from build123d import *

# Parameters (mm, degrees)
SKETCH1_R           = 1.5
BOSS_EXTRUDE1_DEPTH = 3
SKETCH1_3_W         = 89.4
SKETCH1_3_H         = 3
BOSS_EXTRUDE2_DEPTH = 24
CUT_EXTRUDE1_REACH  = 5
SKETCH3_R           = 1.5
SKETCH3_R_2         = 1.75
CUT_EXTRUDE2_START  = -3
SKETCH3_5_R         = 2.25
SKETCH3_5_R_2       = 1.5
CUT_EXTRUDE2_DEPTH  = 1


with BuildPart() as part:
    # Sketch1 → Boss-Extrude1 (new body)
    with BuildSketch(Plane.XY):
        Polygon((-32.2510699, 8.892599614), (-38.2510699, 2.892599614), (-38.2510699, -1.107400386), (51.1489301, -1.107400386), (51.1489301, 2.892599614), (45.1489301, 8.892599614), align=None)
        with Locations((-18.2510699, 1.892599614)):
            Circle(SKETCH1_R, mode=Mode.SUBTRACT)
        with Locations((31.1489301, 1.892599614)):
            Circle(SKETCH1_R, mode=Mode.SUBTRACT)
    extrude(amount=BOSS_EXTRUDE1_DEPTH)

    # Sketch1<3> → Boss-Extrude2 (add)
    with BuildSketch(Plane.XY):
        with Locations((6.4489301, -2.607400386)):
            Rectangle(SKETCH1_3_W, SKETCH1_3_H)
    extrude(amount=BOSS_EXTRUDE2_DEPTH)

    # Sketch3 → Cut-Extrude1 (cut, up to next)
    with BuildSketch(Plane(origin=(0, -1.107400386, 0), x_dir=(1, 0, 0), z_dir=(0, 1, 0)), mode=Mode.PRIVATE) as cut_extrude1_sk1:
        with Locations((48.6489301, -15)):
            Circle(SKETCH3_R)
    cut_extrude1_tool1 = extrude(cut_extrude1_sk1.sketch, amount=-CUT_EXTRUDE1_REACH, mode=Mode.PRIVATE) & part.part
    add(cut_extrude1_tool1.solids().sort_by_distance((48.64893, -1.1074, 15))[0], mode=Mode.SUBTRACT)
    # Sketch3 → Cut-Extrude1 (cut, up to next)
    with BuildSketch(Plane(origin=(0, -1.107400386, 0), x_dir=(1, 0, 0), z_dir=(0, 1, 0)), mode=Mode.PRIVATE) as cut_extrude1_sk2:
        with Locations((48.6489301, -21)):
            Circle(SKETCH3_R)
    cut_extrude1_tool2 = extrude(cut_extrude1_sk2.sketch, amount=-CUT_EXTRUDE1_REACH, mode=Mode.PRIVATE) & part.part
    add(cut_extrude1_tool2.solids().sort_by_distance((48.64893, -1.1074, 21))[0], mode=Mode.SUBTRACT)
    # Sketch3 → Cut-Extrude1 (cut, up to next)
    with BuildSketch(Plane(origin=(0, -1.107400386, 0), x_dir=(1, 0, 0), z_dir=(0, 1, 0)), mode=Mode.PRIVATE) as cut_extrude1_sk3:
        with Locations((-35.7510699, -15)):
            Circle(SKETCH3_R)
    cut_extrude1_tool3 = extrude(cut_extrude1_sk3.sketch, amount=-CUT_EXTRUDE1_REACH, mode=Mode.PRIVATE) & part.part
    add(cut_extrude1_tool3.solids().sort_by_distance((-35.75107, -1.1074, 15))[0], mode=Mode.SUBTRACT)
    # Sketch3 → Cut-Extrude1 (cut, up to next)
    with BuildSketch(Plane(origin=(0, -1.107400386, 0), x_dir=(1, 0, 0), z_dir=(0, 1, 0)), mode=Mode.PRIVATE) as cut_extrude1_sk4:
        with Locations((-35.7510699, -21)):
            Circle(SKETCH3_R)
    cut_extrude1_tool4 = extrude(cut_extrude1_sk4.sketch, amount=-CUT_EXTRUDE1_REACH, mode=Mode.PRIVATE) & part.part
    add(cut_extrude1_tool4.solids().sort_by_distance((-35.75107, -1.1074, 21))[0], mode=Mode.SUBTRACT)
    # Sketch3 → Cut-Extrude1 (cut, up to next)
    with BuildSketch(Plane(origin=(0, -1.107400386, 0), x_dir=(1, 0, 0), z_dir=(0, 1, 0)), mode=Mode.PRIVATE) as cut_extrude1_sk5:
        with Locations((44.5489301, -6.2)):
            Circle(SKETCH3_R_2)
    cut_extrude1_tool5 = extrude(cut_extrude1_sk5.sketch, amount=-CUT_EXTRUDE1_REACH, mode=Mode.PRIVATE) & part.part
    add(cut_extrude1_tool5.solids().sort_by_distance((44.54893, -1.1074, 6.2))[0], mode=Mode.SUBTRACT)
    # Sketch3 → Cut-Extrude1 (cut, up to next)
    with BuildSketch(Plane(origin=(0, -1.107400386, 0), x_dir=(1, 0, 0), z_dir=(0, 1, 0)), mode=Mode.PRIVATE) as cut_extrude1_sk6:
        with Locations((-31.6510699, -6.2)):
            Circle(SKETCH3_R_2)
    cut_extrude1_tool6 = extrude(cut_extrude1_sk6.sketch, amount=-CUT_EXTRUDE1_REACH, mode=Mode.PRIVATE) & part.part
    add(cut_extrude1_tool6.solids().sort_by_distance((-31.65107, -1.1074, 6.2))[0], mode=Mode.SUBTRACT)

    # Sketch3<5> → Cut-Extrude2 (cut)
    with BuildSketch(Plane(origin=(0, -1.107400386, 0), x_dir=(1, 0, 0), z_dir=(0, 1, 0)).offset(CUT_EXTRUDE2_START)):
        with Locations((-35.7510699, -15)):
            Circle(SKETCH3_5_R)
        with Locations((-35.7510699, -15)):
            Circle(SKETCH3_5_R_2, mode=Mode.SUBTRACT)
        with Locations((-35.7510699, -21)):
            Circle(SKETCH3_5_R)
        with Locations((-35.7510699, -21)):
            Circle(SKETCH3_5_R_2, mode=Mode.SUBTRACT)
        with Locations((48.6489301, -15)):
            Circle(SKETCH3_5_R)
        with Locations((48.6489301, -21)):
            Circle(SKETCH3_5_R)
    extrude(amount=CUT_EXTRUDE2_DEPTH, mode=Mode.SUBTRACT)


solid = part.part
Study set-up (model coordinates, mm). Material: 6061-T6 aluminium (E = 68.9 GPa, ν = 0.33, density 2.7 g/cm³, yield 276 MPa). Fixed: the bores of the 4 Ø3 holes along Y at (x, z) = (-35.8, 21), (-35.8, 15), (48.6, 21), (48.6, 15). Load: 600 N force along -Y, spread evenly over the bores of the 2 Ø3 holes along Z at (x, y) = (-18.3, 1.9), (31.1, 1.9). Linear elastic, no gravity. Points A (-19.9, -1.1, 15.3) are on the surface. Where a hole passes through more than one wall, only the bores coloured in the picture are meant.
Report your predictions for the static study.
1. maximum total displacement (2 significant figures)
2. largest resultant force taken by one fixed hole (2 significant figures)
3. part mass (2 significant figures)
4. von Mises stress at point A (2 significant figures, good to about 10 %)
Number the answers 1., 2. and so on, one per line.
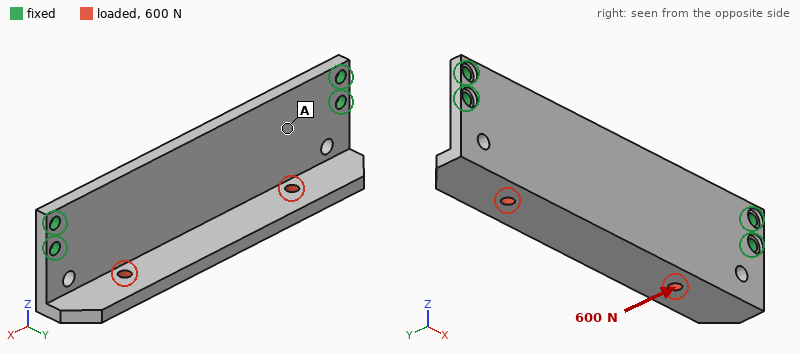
1. 0.26 mm
2. 600 N
3. 24 g
4. 41 MPa
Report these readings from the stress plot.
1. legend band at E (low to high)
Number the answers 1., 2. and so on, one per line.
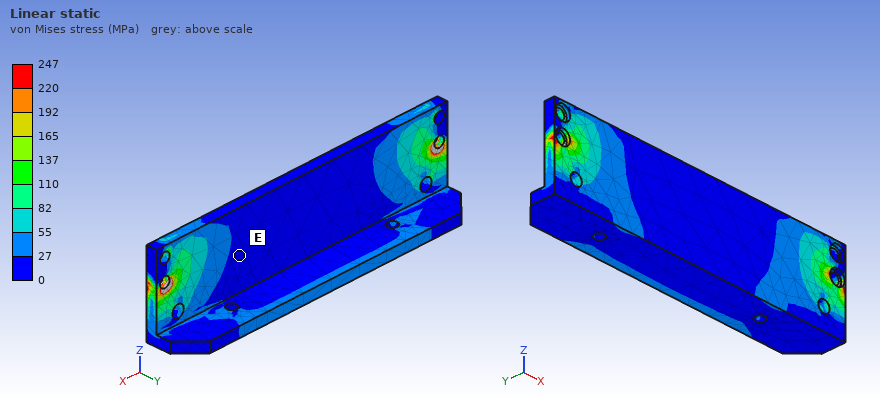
1. 0 to 27 MPa
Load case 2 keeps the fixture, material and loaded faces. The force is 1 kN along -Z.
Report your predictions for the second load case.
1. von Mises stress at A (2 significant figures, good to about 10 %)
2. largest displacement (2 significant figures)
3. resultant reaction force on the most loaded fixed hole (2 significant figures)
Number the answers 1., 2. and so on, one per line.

1. 47 MPa
2. 0.18 mm
3. 440 N
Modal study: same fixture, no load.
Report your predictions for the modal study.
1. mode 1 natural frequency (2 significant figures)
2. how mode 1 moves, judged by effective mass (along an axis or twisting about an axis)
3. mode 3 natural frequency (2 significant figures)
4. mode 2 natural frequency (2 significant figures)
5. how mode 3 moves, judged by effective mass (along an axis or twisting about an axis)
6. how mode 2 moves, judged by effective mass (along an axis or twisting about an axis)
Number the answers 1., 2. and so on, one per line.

1. 2400 Hz
2. along Y
3. 5000 Hz
4. 3300 Hz
5. twisting about Z
6. along Y
